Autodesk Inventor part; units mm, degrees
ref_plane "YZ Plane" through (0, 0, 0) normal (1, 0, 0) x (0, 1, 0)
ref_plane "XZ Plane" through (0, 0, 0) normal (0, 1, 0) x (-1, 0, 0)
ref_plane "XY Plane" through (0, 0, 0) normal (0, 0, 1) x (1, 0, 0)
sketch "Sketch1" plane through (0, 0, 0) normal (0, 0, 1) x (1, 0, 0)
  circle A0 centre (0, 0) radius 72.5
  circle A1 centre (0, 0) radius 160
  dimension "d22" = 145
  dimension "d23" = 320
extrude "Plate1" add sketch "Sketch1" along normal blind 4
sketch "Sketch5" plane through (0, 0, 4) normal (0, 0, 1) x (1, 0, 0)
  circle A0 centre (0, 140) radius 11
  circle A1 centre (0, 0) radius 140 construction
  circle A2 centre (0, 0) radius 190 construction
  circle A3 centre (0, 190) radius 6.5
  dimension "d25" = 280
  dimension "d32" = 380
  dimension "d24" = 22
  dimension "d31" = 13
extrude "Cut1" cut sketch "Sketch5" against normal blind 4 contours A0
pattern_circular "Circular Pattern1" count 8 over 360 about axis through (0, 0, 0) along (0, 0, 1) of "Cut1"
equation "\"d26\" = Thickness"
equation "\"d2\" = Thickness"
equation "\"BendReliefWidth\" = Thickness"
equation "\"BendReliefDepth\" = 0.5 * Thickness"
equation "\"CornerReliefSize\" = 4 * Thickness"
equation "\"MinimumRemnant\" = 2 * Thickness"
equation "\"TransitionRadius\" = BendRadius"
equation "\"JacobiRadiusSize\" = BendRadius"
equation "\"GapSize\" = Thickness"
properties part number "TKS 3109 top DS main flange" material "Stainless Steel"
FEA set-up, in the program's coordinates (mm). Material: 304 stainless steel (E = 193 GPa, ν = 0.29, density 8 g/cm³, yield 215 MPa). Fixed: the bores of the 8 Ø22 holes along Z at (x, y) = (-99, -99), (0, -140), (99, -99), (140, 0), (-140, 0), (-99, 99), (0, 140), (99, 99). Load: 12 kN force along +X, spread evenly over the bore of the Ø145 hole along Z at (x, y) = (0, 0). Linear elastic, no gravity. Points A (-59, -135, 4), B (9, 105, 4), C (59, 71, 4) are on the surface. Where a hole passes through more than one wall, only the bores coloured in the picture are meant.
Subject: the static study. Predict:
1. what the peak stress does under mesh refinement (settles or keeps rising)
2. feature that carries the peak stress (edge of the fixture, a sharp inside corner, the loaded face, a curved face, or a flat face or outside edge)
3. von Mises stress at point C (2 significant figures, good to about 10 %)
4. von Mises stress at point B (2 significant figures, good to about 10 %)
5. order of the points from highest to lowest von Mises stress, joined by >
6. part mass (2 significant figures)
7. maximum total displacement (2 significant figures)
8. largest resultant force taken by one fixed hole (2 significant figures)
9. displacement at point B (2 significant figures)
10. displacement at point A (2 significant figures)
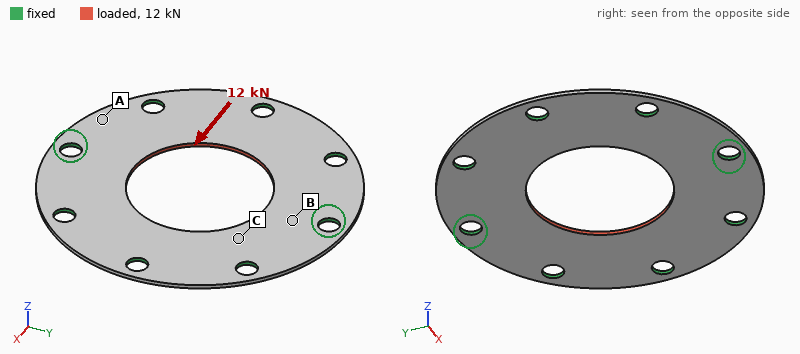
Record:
keeps rising
edge of the fixture
7.4 MPa
4.2 MPa
C > B > A
1.9 kg
3.2 µm
2.2 kN
1.2 µm
0.67 µm
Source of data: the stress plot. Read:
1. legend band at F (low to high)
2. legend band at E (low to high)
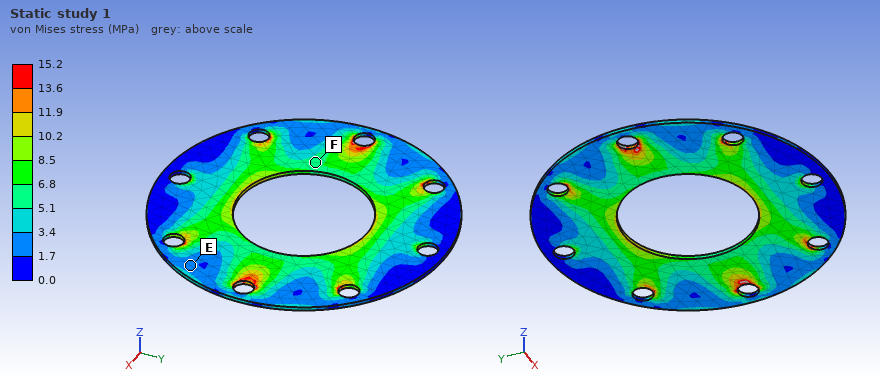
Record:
5.1 to 6.8 MPa
1.7 to 3.4 MPa
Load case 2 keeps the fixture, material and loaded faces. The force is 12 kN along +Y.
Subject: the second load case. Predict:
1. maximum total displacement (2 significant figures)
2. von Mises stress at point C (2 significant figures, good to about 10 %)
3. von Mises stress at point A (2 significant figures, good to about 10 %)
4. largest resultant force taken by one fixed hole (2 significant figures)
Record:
3.2 µm
5.9 MPa
2.3 MPa
2.2 kN
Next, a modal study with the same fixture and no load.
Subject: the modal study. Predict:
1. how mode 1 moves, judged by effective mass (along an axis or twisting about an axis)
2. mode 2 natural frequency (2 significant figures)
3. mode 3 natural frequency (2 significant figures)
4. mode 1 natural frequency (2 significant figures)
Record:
along Z
1100 Hz
1100 Hz
950 Hz
